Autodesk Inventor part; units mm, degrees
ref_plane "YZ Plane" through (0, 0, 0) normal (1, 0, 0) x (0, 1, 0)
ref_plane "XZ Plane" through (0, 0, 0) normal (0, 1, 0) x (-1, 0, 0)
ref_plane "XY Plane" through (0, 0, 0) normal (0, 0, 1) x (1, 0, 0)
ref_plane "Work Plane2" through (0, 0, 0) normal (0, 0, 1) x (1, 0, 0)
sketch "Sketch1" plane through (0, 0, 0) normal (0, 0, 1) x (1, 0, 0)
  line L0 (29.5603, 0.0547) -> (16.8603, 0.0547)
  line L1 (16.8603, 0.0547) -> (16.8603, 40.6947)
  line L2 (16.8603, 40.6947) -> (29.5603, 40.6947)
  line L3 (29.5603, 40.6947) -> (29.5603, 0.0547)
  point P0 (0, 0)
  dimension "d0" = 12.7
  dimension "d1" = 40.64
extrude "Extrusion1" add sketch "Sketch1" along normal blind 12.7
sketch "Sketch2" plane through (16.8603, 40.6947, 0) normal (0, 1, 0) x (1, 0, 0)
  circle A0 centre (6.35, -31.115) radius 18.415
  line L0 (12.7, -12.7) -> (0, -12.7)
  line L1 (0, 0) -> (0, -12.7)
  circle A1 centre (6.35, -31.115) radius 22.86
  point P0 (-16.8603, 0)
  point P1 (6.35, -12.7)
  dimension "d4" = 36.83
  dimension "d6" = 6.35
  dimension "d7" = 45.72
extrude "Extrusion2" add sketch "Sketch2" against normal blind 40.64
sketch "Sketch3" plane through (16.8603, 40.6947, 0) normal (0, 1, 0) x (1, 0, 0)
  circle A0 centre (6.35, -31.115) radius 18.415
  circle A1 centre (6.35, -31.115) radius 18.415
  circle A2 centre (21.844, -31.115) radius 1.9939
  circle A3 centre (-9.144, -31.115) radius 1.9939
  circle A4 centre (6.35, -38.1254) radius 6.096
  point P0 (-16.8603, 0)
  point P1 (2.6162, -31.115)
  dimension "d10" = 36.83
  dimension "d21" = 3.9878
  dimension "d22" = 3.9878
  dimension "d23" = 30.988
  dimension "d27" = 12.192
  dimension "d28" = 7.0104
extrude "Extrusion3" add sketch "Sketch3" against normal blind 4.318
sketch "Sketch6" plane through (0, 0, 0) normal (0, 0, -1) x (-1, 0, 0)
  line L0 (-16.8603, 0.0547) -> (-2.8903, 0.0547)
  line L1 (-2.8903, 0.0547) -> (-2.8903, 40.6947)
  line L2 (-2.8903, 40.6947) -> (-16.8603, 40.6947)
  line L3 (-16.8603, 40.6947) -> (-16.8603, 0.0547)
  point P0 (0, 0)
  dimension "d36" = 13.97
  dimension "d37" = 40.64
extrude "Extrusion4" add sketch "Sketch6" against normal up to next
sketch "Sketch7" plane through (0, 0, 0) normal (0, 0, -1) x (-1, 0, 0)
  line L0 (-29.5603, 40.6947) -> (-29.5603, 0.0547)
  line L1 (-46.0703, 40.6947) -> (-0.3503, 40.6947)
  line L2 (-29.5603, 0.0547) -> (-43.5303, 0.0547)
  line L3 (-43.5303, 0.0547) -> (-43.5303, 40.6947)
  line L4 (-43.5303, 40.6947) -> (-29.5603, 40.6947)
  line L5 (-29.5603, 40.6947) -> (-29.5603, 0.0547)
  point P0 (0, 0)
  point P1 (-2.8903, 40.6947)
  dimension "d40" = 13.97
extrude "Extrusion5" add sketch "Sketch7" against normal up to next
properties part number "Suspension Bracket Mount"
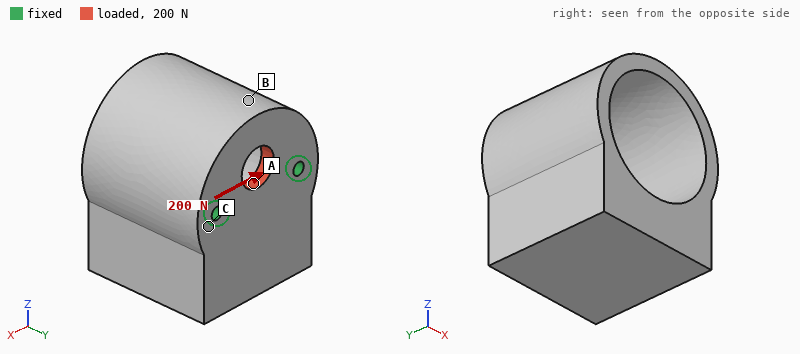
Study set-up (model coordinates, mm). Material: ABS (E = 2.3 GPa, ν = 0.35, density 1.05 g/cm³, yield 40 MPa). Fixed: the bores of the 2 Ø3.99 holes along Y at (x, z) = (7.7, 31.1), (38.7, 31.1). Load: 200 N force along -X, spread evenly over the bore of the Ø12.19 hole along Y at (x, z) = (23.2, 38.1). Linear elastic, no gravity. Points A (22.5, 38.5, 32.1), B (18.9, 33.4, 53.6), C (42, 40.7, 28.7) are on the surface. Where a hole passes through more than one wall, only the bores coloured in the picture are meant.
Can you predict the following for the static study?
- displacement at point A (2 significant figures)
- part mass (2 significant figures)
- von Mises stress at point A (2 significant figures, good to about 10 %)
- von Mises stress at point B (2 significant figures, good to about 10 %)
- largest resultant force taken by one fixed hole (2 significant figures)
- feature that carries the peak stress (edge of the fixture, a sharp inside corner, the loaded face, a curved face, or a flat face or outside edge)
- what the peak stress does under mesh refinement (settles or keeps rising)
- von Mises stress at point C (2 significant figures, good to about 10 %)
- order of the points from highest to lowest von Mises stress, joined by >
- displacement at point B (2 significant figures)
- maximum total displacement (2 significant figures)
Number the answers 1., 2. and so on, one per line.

1. 7.4 µm
2. 49 g
3. 2.1 MPa
4. 0.33 MPa
5. 110 N
6. edge of the fixture
7. keeps rising
8. 0.88 MPa
9. A > C > B
10. 18 µm
11. 24 µm
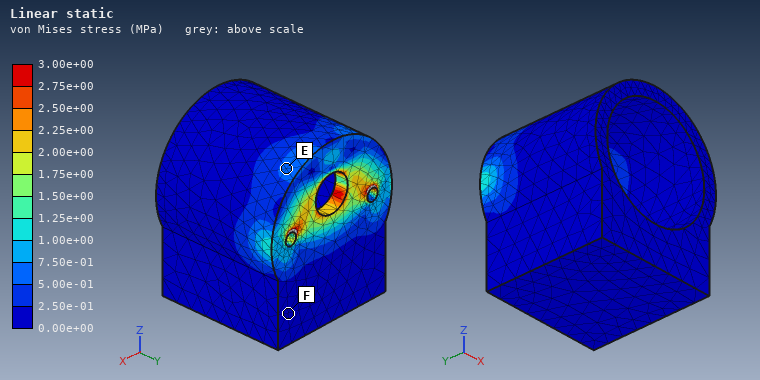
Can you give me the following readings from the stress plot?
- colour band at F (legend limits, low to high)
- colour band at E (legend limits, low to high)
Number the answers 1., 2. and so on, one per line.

1. 0.00e+00 to 2.50e-01 MPa
2. 5.00e-01 to 7.50e-01 MPa
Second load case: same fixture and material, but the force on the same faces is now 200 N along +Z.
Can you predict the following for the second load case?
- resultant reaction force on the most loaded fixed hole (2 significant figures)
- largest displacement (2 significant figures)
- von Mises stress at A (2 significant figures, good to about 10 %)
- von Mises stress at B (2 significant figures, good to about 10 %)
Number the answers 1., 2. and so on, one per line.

1. 100 N
2. 18 µm
3. 1.1 MPa
4. 0.58 MPa
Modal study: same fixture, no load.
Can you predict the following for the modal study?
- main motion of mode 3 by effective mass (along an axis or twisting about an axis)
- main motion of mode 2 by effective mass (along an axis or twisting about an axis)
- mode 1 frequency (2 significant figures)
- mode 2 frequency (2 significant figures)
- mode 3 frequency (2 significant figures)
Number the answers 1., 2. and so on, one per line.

1. along Y
2. along X
3. 410 Hz
4. 1300 Hz
5. 2400 Hz
